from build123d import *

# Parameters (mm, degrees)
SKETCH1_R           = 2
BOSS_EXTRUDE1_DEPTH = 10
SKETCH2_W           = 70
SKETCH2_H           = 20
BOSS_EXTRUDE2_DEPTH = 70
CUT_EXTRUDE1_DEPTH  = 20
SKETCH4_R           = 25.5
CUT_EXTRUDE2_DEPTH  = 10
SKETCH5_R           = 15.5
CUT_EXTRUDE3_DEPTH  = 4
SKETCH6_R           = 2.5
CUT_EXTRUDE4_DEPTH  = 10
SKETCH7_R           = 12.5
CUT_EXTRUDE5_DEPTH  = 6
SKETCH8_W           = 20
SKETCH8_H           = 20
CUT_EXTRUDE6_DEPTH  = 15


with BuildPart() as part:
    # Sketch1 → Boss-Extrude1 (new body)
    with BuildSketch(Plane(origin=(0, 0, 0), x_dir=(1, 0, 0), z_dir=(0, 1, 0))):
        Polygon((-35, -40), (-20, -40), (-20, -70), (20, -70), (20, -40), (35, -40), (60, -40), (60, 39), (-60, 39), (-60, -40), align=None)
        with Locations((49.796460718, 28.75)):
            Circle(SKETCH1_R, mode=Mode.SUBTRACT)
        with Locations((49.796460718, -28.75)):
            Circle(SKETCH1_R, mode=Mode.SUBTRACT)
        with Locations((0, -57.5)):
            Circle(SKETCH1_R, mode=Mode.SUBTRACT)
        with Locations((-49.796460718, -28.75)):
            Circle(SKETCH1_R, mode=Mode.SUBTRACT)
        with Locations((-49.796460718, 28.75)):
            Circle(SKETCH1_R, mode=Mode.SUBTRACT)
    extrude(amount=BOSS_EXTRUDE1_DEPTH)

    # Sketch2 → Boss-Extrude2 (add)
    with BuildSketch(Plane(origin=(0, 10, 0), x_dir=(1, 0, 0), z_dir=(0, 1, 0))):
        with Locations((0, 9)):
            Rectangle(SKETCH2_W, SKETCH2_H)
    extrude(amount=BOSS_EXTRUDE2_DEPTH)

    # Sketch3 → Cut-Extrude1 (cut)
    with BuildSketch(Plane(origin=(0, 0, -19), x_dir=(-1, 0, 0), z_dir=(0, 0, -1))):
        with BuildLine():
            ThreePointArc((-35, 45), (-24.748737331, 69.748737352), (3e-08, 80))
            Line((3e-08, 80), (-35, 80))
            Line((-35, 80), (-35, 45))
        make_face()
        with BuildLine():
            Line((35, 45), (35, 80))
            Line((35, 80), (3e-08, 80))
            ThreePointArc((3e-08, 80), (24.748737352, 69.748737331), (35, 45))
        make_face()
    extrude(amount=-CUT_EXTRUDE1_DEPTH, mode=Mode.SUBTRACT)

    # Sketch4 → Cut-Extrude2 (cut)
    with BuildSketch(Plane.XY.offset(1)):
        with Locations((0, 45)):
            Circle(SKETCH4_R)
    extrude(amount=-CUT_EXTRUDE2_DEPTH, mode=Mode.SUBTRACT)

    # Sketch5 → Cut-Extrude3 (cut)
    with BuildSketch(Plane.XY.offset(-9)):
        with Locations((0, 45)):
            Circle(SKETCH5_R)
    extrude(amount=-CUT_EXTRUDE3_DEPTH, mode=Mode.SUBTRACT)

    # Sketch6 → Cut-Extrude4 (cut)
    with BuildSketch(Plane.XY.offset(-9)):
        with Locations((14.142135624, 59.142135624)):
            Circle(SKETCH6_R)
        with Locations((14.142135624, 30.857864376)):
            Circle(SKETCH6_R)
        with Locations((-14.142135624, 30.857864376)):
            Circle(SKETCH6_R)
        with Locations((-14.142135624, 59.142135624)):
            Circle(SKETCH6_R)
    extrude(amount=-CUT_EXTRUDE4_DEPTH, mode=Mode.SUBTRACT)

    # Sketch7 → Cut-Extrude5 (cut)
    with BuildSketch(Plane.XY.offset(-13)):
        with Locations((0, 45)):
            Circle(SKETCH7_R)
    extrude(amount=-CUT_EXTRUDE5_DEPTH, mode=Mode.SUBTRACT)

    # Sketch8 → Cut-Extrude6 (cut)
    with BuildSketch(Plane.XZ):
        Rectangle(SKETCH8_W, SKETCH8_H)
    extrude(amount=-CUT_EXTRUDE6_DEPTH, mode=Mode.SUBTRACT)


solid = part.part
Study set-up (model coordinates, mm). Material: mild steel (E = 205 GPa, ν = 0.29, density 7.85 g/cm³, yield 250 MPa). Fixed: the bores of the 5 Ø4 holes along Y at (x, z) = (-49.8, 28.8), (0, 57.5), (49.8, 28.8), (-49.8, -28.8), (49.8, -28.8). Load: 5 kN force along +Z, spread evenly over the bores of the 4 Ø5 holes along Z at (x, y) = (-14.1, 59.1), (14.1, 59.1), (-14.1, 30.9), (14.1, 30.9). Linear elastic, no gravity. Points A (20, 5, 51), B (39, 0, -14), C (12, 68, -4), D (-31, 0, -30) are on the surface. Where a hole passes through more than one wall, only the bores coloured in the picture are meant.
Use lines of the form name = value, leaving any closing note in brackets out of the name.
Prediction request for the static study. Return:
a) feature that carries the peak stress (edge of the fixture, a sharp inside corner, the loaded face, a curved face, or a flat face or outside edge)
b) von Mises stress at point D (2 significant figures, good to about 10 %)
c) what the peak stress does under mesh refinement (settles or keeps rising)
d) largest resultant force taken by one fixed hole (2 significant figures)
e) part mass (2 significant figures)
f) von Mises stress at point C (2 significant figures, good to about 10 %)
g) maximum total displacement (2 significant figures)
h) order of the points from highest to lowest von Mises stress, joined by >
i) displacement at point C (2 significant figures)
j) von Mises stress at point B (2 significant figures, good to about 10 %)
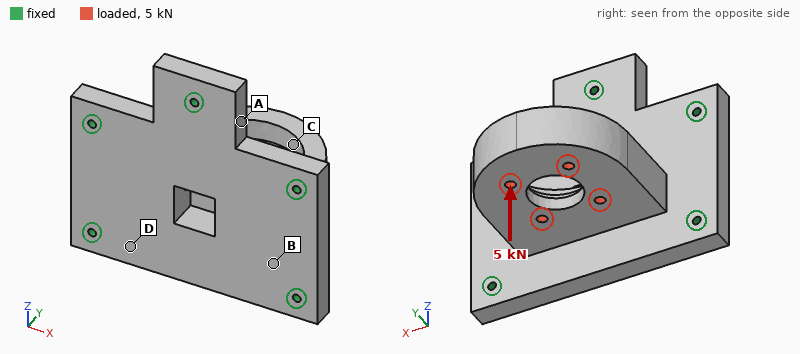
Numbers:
feature that carries the peak stress = edge of the fixture
von Mises stress at point D = 23 MPa
what the peak stress does under mesh refinement = keeps rising
largest resultant force taken by one fixed hole = 2.2 kN
part mass = 1.3 kg
von Mises stress at point C = 14 MPa
maximum total displacement = 0.11 mm
order of the points from highest to lowest von Mises stress, joined by > = B > D > C > A
displacement at point C = 0.087 mm
von Mises stress at point B = 34 MPa
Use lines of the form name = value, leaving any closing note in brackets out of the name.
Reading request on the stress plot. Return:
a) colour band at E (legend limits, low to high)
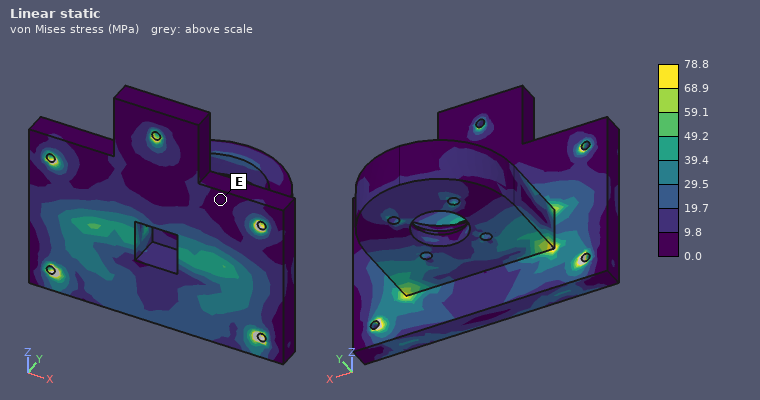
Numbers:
colour band at E = 0.0 to 9.8 MPa
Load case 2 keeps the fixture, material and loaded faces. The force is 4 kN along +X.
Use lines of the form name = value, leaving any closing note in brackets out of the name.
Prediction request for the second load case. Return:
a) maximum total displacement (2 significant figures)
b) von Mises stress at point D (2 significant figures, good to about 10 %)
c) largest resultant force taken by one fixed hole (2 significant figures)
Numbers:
maximum total displacement = 18 µm
von Mises stress at point D = 7.4 MPa
largest resultant force taken by one fixed hole = 1.8 kN
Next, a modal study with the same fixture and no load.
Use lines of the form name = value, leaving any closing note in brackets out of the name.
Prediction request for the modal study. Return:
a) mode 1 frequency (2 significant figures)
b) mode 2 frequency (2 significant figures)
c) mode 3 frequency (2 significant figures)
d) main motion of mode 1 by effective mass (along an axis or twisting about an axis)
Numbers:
mode 1 frequency = 2100 Hz
mode 2 frequency = 4000 Hz
mode 3 frequency = 4100 Hz
main motion of mode 1 by effective mass = along Z
